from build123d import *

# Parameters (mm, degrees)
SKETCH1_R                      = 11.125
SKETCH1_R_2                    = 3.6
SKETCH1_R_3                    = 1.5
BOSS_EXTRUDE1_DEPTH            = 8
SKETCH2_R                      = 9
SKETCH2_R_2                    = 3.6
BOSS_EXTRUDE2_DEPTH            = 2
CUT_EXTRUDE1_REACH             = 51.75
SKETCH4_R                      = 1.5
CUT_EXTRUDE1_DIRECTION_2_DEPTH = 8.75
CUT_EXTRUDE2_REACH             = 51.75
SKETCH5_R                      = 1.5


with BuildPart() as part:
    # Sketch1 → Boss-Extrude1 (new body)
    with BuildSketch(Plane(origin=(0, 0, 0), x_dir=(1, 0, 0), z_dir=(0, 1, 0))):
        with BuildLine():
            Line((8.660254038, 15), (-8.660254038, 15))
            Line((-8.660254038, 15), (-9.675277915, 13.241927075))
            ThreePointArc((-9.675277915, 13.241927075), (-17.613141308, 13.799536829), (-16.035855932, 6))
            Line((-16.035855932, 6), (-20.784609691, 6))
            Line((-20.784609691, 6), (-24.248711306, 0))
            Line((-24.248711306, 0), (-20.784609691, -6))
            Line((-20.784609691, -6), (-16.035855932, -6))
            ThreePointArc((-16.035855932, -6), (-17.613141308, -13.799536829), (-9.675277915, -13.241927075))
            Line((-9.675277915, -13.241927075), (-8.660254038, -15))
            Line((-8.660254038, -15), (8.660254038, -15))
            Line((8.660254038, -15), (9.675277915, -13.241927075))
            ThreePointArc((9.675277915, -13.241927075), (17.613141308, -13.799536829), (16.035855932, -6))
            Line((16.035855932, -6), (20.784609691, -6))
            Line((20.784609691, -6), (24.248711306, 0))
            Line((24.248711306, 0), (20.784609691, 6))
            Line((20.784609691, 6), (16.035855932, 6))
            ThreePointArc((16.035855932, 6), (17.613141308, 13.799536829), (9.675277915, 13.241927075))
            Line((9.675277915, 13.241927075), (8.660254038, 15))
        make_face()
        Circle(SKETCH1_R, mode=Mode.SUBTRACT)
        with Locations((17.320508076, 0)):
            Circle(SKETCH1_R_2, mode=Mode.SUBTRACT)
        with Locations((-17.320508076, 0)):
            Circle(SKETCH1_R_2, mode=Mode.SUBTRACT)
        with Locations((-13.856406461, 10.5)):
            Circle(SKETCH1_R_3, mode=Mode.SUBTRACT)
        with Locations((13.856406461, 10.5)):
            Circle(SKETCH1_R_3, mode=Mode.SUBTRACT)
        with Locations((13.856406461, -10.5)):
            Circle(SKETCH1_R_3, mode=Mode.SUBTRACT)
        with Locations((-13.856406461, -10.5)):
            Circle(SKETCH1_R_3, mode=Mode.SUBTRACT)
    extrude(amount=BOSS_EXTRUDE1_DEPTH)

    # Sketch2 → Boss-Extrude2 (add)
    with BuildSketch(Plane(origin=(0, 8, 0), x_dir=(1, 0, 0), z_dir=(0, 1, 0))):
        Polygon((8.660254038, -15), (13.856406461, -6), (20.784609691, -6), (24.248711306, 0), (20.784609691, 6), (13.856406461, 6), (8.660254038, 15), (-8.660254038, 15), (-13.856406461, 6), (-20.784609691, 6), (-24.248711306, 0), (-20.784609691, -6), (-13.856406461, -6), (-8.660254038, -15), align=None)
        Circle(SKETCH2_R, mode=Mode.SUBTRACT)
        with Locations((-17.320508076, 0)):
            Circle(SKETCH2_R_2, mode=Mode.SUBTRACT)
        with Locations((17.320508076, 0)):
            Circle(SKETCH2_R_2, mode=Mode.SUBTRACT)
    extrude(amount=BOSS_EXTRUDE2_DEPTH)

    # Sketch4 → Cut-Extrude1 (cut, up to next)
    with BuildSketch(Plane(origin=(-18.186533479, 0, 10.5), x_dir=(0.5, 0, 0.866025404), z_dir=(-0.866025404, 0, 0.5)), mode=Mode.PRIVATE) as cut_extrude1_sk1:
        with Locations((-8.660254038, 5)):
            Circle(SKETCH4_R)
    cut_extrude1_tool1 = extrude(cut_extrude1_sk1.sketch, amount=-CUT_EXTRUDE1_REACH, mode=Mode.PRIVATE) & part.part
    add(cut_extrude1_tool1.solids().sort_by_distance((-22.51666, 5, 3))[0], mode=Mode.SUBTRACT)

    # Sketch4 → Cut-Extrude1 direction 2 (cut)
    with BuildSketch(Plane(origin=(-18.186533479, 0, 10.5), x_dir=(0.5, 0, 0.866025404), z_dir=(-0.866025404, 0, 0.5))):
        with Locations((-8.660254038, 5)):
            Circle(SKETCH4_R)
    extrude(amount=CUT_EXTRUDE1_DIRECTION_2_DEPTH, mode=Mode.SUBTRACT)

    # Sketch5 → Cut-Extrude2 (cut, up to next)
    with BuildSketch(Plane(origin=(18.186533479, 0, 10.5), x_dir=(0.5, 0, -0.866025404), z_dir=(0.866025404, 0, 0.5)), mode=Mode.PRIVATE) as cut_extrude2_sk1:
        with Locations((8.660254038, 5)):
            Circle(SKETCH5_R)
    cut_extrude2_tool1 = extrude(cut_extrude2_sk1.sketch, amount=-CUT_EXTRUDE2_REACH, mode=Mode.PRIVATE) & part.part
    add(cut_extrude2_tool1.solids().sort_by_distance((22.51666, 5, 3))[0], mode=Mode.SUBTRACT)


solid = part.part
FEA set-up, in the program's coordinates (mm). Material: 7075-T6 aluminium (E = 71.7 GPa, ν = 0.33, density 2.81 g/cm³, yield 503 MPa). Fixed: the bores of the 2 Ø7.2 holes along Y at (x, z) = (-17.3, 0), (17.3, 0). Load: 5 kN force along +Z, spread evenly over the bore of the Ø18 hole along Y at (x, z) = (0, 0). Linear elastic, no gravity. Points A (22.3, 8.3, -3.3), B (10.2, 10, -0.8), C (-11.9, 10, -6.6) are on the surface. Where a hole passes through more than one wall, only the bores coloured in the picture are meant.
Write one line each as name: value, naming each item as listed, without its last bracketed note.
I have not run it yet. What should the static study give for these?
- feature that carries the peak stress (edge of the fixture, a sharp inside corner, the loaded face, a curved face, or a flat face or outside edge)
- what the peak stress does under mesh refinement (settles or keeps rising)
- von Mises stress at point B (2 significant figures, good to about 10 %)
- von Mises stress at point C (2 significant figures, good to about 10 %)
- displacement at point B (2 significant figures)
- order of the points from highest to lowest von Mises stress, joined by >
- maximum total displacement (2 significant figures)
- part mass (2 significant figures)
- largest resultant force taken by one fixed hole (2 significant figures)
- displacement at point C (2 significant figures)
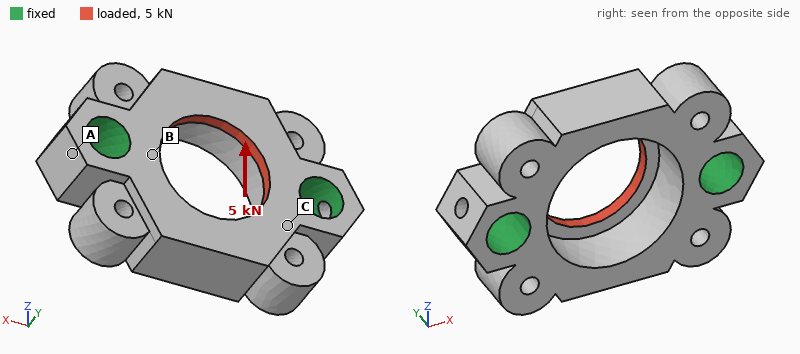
feature that carries the peak stress: edge of the fixture
what the peak stress does under mesh refinement: keeps rising
von Mises stress at point B: 70 MPa
von Mises stress at point C: 54 MPa
displacement at point B: 7.2 µm
order of the points from highest to lowest von Mises stress, joined by >: B > C > A
maximum total displacement: 23 µm
part mass: 19 g
largest resultant force taken by one fixed hole: 2.5 kN
displacement at point C: 7.1 µm
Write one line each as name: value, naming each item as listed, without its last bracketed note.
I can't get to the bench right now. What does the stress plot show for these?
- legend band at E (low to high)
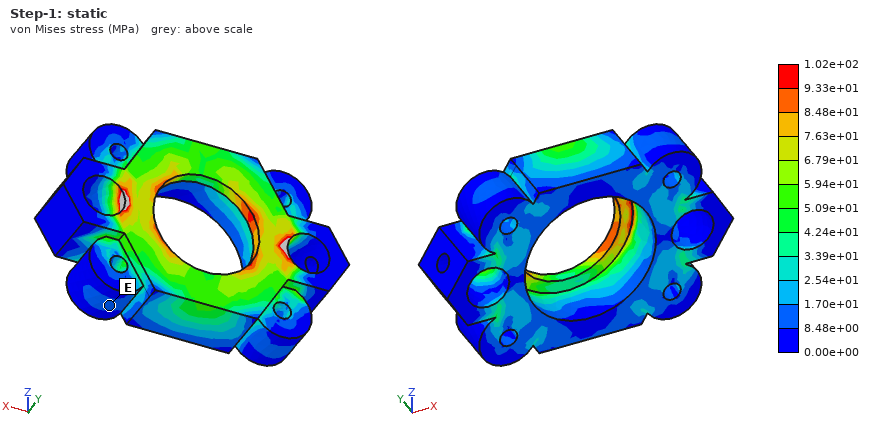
legend band at E: 8.48e+00 to 1.70e+01 MPa
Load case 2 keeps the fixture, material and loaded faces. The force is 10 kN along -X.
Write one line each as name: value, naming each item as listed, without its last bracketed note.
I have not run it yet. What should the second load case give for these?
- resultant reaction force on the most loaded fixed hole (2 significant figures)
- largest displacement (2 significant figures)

resultant reaction force on the most loaded fixed hole: 5.0 kN
largest displacement: 27 µm
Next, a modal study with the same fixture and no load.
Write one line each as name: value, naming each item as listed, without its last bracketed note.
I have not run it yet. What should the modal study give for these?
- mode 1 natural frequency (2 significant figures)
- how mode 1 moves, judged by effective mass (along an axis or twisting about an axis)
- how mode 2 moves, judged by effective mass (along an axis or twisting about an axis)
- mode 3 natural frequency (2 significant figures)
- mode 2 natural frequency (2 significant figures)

mode 1 natural frequency: 21 kHz
how mode 1 moves, judged by effective mass: twisting about X
how mode 2 moves, judged by effective mass: along Y
mode 3 natural frequency: 29 kHz
mode 2 natural frequency: 23 kHz
